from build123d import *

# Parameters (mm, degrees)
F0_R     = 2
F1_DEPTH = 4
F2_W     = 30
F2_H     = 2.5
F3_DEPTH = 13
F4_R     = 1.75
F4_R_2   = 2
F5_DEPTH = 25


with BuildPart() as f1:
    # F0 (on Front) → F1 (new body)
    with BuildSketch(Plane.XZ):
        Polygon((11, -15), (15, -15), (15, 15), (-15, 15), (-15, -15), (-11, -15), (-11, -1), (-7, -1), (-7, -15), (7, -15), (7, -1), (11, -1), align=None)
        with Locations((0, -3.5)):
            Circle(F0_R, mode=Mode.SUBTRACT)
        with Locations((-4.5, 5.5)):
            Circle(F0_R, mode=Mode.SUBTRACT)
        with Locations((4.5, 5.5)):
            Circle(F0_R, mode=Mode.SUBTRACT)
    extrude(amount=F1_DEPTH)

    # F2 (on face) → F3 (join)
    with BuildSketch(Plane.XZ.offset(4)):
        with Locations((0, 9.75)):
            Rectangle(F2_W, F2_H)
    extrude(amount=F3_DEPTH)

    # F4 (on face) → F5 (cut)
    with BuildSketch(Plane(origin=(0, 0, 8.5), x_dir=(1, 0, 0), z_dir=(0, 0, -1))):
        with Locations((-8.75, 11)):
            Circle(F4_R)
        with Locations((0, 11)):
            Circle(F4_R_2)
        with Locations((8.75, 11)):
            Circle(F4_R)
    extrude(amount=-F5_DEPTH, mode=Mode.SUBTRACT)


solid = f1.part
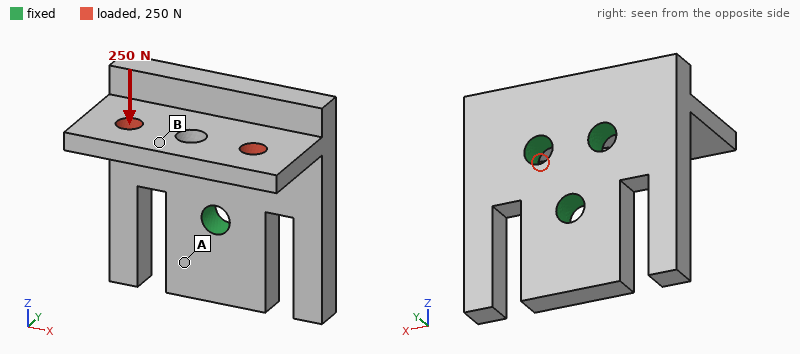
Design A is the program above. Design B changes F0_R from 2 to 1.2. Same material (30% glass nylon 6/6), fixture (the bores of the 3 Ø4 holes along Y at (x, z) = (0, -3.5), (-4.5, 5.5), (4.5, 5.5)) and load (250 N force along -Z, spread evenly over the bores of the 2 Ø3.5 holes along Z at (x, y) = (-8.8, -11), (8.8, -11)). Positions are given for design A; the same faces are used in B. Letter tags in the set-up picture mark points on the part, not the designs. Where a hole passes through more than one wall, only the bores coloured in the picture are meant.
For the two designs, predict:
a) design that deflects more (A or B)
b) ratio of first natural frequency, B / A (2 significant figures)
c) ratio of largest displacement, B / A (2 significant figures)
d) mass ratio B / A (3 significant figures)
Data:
B
0.94
1.1
1.02
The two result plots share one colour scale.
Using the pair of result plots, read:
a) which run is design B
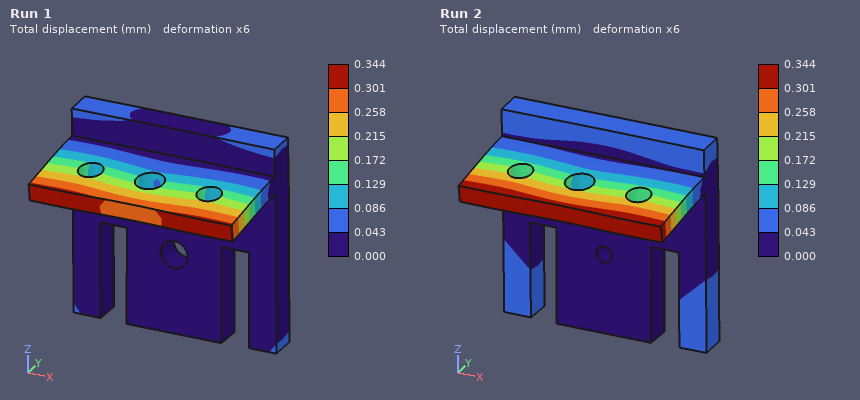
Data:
Run 2
